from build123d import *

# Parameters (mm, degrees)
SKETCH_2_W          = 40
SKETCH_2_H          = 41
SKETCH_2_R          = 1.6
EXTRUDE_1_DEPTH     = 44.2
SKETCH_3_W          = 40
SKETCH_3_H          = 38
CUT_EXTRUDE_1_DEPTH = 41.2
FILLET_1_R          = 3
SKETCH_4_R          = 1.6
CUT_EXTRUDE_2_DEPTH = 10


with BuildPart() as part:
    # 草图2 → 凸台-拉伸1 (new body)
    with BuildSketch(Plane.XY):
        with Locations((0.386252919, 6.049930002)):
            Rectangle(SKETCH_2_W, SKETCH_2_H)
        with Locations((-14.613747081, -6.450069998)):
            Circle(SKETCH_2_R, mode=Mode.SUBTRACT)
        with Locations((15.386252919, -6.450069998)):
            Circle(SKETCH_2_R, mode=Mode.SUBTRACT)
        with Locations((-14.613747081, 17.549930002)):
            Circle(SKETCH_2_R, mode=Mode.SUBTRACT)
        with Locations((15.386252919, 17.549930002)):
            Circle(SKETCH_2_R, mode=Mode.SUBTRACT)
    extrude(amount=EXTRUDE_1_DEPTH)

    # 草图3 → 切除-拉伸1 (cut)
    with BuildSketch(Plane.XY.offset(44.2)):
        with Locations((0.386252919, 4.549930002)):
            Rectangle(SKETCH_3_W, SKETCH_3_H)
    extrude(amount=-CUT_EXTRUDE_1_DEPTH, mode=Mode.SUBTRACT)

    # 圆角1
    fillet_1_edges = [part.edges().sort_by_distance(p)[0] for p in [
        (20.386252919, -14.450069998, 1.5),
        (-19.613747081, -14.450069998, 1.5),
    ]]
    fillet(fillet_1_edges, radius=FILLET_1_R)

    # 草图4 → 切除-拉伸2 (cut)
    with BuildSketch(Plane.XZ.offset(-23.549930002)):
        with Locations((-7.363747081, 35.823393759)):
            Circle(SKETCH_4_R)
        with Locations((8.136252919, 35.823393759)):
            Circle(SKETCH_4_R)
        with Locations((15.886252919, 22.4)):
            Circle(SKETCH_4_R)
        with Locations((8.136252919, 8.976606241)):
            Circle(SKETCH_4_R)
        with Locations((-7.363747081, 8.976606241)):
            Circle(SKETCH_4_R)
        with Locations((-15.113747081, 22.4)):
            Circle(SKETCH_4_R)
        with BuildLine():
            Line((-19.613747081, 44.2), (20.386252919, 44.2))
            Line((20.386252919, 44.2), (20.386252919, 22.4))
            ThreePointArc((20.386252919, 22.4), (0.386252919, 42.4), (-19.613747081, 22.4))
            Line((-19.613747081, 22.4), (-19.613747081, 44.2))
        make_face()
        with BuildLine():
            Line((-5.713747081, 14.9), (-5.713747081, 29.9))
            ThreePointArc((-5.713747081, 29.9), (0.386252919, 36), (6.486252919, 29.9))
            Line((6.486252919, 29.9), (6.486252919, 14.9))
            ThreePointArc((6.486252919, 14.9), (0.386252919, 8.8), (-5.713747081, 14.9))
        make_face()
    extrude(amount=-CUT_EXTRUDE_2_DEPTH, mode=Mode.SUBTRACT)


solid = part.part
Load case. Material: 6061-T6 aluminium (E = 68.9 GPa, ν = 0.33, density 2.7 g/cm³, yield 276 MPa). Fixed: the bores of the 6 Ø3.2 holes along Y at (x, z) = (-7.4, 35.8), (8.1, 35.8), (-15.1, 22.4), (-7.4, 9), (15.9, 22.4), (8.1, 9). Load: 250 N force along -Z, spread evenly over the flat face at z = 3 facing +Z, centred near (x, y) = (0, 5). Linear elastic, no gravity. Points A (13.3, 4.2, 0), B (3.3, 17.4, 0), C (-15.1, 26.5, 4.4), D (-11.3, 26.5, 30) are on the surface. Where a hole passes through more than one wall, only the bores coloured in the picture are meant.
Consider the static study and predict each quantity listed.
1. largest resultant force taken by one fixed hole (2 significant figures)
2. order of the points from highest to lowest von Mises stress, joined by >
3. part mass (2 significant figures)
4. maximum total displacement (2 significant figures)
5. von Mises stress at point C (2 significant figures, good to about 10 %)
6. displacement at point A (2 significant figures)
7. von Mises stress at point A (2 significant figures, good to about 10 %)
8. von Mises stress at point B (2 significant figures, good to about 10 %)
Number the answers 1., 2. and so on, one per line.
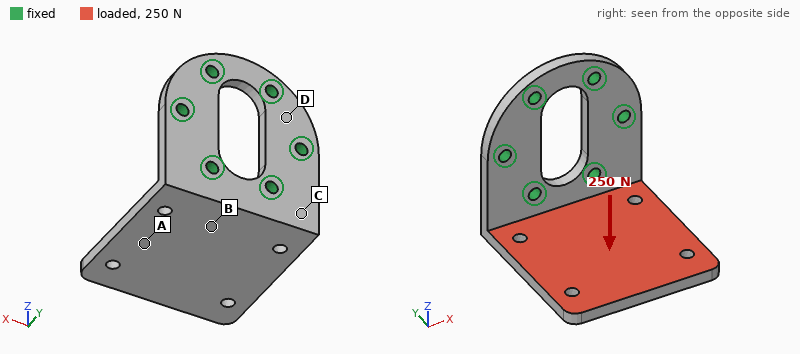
1. 130 N
2. C > B > A > D
3. 22 g
4. 0.54 mm
5. 64 MPa
6. 0.24 mm
7. 19 MPa
8. 53 MPa
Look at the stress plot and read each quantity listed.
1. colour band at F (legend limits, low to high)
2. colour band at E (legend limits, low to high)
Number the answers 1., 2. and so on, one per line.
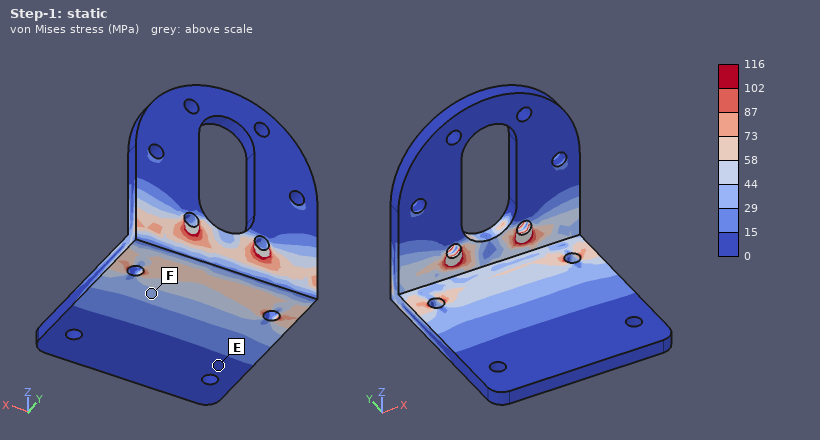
1. 29 to 44 MPa
2. 0 to 15 MPa
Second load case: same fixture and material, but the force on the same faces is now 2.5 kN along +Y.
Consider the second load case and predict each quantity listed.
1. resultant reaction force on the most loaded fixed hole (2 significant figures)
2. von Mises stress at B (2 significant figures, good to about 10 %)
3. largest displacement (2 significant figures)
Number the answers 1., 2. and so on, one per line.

1. 1.3 kN
2. 34 MPa
3. 96 µm
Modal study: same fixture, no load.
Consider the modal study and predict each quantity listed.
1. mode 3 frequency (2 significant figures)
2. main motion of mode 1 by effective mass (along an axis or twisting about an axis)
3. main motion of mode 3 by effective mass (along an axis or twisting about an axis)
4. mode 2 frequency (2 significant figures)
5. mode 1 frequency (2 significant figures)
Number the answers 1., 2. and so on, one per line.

1. 4300 Hz
2. along Z
3. along X
4. 3100 Hz
5. 1200 Hz
